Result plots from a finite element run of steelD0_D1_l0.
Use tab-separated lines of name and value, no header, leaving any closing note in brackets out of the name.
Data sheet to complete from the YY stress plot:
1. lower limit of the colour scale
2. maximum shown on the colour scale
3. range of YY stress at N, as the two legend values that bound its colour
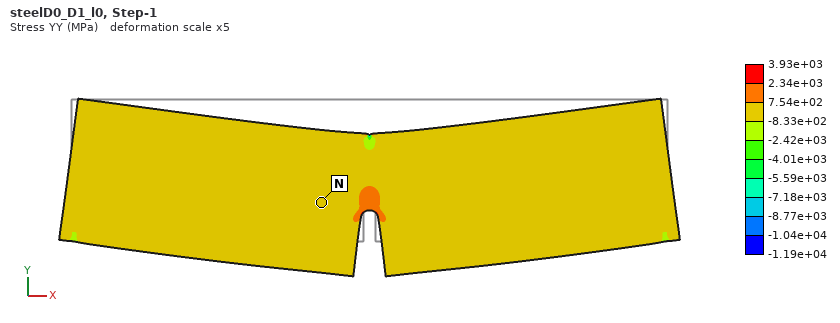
lower limit of the colour scale	-1.19e+04 MPa
maximum shown on the colour scale	3.93e+03 MPa
range of YY stress at N, as the two legend values that bound its colour	-8.33e+02 to 7.54e+02 MPa
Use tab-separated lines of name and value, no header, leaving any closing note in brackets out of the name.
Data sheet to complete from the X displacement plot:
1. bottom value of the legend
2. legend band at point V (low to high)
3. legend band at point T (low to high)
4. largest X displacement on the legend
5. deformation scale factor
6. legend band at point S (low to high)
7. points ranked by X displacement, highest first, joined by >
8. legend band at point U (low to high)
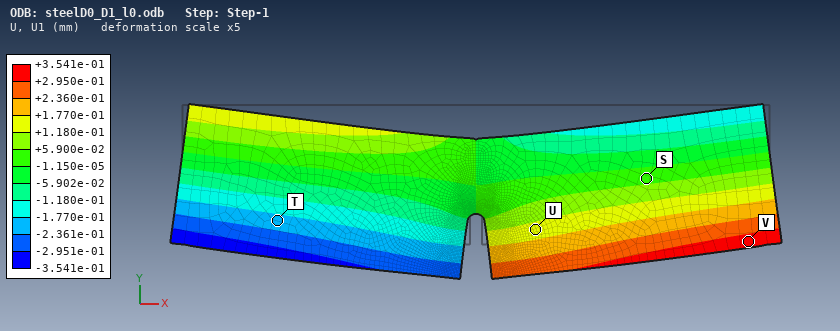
bottom value of the legend	-3.541e-01 mm
legend band at point V	+2.950e-01 to +3.541e-01 mm
legend band at point T	-2.361e-01 to -1.770e-01 mm
largest X displacement on the legend	+3.541e-01 mm
deformation scale factor	5
legend band at point S	-1.150e-05 to +5.900e-02 mm
points ranked by X displacement, highest first, joined by >	V > U > S > T
legend band at point U	+1.180e-01 to +1.770e-01 mm
